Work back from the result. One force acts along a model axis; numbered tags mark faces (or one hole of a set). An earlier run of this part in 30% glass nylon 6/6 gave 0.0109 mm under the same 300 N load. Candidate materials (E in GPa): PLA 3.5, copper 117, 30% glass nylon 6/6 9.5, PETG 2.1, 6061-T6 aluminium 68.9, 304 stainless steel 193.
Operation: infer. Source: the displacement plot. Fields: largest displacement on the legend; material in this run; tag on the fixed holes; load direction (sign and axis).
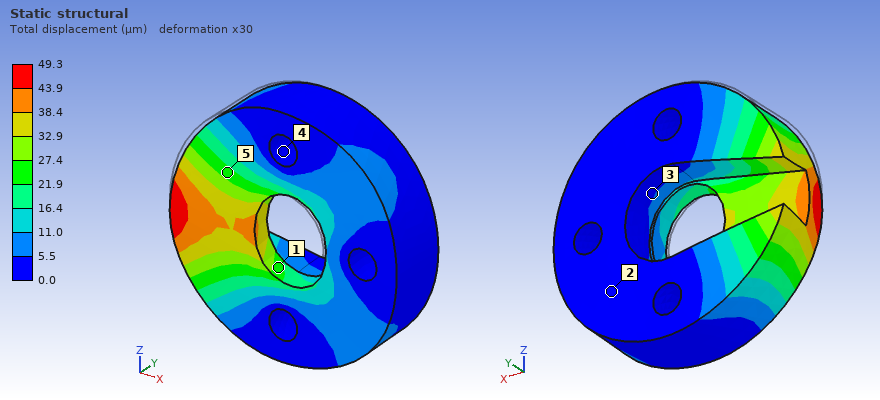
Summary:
49.3 µm
PETG
4
+X
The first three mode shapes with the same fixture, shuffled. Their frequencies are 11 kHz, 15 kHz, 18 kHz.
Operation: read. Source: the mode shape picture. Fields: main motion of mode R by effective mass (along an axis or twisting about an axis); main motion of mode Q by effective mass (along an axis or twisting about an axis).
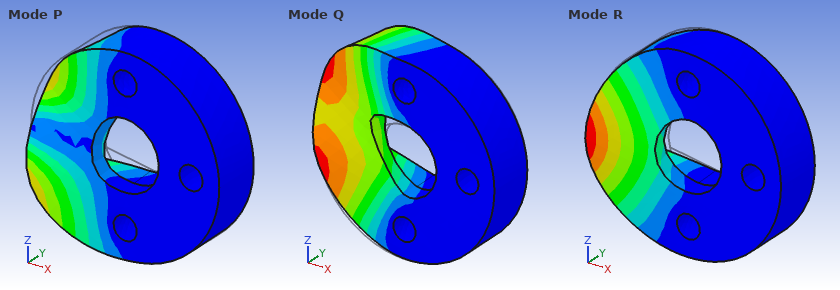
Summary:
along Y
along Z
